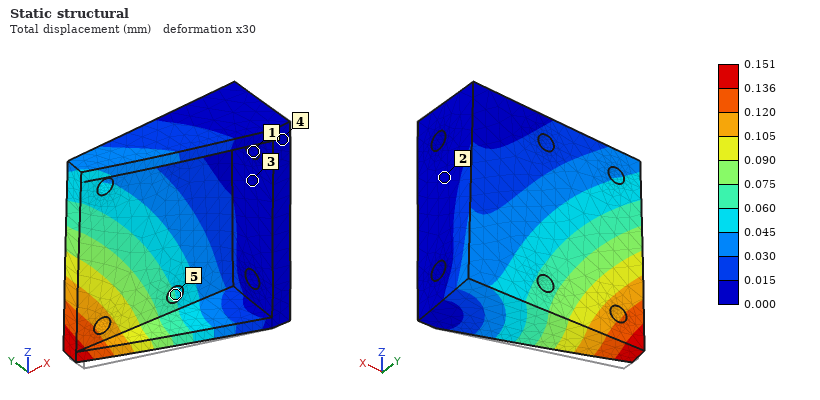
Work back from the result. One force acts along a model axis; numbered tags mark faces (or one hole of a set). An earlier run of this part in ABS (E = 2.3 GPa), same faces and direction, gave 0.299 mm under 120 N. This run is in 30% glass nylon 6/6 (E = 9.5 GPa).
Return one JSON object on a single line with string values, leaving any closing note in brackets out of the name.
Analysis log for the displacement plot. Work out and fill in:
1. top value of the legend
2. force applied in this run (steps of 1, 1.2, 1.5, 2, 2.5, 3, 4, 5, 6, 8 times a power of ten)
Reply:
{"top value of the legend": "0.151 mm", "force applied in this run": "250 N"}
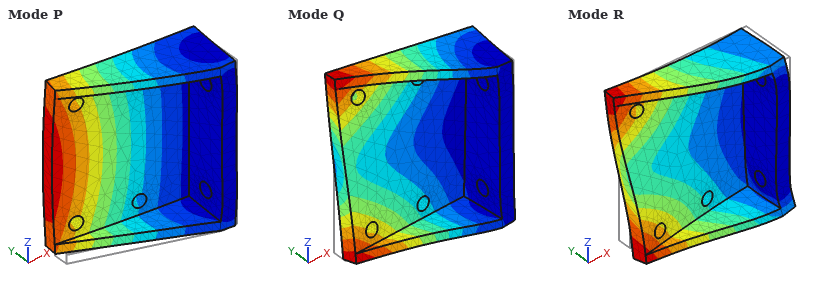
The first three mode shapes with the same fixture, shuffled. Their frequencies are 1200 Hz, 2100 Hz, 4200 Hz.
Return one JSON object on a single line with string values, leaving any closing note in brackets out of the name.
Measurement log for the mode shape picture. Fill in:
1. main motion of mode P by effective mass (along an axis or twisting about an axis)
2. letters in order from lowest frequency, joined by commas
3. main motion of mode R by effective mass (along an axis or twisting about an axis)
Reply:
{"main motion of mode P by effective mass": "along Y", "letters in order from lowest frequency, joined by commas": "P, Q, R", "main motion of mode R by effective mass": "along Z"}
